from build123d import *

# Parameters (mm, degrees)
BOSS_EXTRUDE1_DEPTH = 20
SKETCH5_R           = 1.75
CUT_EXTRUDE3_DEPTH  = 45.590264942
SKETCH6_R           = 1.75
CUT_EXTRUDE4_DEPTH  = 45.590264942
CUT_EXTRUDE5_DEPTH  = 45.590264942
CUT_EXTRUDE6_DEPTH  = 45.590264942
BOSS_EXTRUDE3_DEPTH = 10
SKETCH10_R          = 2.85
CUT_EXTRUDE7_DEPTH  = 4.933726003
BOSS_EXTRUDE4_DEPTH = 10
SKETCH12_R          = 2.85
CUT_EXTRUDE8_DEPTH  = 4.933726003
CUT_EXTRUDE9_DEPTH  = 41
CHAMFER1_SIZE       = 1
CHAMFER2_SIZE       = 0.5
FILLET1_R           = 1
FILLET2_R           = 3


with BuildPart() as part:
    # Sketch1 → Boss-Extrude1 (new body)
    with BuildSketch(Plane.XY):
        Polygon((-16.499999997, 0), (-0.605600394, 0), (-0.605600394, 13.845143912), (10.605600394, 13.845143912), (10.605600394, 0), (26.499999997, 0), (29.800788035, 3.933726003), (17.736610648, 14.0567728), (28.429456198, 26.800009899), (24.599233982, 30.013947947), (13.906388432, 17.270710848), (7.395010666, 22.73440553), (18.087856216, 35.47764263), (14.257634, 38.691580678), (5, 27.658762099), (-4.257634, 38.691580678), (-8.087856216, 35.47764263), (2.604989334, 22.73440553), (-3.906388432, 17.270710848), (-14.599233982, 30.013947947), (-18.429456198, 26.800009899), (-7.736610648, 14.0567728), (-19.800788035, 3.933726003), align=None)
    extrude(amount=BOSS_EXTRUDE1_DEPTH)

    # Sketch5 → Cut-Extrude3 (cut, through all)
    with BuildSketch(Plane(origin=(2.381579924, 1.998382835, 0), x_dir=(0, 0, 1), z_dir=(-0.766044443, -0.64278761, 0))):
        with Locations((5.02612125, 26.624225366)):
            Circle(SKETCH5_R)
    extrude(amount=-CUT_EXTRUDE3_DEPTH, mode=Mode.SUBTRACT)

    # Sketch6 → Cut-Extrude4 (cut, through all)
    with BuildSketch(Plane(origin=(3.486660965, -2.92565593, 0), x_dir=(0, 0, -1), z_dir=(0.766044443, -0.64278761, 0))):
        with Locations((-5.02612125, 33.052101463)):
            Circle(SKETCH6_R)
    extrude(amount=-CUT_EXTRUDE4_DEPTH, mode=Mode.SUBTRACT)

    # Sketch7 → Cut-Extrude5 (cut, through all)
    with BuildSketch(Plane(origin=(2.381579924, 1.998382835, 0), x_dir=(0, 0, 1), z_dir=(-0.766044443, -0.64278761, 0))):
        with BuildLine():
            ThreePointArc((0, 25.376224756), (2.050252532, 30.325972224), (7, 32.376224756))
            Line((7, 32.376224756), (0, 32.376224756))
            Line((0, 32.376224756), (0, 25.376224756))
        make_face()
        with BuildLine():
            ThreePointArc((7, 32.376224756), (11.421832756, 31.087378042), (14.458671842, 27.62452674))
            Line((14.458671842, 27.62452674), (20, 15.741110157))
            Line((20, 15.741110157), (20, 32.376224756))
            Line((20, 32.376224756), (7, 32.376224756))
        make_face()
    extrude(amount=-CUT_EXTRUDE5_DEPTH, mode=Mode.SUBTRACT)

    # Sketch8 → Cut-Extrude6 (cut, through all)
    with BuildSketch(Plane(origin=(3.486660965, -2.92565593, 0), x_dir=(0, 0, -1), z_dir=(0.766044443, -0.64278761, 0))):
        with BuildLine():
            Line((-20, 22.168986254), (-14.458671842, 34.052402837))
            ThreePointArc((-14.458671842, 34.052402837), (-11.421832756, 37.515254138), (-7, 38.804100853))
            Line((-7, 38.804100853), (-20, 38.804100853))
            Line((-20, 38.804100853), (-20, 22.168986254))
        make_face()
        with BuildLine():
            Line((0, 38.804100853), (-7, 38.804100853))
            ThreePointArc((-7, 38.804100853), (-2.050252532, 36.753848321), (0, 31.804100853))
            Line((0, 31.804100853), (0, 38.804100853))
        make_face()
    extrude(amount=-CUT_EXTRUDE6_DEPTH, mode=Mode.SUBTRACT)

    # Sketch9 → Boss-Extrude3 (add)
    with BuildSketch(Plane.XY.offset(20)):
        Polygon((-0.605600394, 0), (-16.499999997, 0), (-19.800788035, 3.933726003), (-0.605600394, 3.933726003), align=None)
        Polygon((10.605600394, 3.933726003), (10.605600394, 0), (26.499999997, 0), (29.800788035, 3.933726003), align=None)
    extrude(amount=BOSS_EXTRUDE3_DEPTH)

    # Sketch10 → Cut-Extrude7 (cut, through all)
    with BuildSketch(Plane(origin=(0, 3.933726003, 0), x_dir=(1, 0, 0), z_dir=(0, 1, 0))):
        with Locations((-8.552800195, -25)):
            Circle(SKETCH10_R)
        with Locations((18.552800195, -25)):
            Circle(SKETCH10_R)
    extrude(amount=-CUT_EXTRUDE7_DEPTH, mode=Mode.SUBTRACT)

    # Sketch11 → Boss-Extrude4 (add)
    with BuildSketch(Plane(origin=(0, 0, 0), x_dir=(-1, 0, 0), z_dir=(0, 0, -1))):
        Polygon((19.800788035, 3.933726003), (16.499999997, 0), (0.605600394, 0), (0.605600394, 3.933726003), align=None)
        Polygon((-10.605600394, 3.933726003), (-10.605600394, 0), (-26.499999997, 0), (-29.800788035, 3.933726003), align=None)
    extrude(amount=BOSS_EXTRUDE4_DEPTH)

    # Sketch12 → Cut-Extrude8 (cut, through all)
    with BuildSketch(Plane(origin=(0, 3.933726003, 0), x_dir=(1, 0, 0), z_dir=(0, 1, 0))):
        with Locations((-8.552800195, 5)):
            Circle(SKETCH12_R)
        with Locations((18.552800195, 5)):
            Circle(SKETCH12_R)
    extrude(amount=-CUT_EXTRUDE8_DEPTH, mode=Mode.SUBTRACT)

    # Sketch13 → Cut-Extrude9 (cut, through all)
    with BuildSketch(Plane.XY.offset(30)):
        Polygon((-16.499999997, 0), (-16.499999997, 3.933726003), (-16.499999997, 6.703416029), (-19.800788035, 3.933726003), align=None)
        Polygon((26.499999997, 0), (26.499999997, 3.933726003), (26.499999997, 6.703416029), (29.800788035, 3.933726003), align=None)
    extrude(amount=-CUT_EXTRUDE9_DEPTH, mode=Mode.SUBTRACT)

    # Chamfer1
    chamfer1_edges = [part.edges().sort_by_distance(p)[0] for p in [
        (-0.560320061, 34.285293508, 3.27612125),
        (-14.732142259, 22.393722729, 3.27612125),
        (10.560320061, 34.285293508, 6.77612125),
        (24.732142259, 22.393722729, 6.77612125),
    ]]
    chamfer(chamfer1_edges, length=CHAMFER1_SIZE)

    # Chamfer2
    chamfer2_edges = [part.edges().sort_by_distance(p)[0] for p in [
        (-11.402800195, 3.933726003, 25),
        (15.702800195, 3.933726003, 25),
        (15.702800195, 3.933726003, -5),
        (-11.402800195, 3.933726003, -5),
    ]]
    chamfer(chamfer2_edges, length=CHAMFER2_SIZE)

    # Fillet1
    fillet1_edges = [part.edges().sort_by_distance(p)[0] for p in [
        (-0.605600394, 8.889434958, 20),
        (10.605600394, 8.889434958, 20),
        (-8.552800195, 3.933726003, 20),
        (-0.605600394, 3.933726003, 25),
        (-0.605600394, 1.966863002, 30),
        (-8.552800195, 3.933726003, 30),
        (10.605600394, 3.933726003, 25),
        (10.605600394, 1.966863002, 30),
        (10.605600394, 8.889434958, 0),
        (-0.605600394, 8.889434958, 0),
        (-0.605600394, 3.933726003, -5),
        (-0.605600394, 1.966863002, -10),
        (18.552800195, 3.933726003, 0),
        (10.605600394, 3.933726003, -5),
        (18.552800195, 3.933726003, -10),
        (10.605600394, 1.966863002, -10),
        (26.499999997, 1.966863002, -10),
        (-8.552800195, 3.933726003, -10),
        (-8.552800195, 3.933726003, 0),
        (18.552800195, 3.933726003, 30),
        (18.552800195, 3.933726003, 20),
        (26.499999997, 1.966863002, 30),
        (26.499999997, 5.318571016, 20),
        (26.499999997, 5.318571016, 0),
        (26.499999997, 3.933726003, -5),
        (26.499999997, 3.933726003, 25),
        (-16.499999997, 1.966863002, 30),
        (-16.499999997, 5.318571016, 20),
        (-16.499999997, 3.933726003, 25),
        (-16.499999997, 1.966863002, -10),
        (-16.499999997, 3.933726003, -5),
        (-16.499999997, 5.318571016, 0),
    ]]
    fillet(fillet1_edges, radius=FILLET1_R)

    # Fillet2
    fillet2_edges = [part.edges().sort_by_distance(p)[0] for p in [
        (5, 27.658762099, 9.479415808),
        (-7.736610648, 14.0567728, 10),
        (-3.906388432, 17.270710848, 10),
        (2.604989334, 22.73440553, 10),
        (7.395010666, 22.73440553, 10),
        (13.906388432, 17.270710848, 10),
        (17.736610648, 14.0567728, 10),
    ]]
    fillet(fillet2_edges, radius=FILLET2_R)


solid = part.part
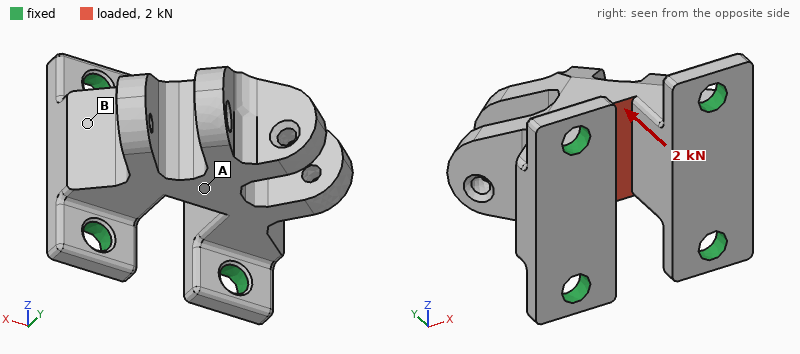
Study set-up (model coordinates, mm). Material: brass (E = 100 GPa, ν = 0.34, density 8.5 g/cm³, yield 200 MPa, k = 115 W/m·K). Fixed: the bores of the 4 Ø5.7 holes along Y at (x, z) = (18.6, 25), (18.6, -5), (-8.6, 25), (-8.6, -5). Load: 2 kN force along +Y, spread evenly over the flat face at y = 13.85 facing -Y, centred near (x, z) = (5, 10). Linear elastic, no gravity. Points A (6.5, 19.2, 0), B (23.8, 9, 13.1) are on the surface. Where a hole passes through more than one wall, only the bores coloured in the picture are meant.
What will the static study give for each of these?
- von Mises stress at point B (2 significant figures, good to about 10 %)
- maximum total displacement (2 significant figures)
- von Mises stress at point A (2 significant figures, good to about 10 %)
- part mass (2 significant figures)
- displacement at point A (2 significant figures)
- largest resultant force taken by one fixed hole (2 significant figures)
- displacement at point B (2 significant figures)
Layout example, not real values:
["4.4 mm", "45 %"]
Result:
["4.2 MPa", "5.5 µm", "13 MPa", "150 g", "5.0 µm", "610 N", "2.4 µm"]
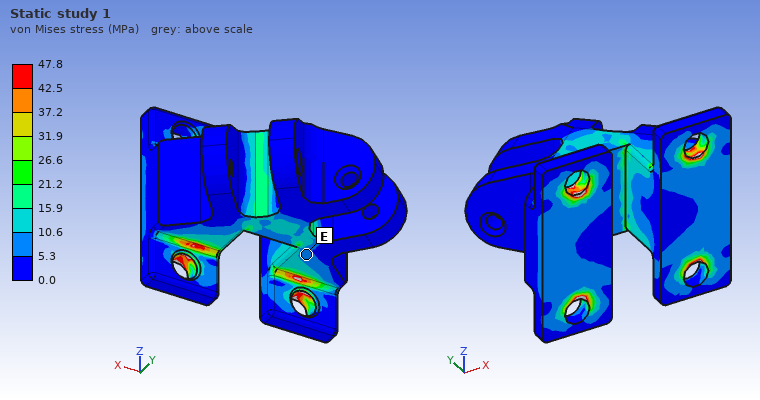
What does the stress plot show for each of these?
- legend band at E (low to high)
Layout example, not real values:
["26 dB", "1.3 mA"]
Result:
["5.3 to 10.6 MPa"]
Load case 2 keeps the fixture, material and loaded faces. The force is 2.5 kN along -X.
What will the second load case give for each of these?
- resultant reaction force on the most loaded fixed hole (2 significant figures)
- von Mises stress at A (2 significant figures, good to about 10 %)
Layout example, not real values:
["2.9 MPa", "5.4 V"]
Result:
["740 N", "17 MPa"]
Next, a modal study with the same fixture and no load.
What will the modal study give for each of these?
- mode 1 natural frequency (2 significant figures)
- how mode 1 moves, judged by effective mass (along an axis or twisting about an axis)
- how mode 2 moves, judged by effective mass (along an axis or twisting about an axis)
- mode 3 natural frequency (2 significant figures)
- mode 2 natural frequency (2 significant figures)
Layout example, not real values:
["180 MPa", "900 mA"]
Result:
["6300 Hz", "along X", "along Z", "8100 Hz", "6600 Hz"]
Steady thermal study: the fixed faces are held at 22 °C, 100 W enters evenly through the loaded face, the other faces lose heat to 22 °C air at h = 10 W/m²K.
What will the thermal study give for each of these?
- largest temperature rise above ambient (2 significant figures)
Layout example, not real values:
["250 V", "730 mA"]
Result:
["73 K"]
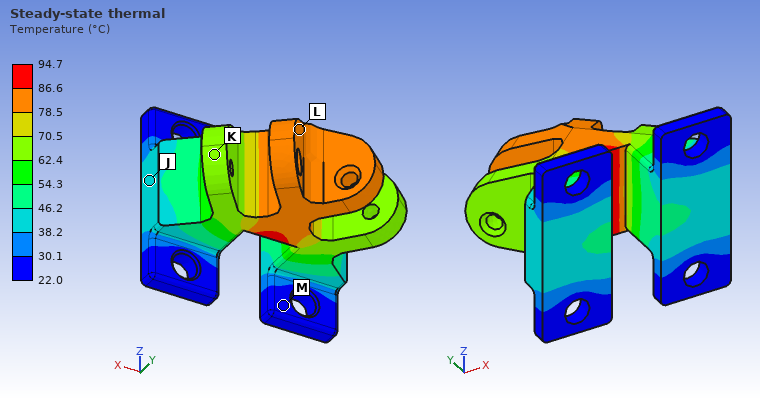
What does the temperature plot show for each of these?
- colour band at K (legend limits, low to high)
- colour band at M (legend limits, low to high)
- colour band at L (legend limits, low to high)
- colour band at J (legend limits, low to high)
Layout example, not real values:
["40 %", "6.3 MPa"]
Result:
["62.4 to 70.5 °C", "22.0 to 30.1 °C", "78.5 to 86.6 °C", "38.2 to 46.2 °C"]
